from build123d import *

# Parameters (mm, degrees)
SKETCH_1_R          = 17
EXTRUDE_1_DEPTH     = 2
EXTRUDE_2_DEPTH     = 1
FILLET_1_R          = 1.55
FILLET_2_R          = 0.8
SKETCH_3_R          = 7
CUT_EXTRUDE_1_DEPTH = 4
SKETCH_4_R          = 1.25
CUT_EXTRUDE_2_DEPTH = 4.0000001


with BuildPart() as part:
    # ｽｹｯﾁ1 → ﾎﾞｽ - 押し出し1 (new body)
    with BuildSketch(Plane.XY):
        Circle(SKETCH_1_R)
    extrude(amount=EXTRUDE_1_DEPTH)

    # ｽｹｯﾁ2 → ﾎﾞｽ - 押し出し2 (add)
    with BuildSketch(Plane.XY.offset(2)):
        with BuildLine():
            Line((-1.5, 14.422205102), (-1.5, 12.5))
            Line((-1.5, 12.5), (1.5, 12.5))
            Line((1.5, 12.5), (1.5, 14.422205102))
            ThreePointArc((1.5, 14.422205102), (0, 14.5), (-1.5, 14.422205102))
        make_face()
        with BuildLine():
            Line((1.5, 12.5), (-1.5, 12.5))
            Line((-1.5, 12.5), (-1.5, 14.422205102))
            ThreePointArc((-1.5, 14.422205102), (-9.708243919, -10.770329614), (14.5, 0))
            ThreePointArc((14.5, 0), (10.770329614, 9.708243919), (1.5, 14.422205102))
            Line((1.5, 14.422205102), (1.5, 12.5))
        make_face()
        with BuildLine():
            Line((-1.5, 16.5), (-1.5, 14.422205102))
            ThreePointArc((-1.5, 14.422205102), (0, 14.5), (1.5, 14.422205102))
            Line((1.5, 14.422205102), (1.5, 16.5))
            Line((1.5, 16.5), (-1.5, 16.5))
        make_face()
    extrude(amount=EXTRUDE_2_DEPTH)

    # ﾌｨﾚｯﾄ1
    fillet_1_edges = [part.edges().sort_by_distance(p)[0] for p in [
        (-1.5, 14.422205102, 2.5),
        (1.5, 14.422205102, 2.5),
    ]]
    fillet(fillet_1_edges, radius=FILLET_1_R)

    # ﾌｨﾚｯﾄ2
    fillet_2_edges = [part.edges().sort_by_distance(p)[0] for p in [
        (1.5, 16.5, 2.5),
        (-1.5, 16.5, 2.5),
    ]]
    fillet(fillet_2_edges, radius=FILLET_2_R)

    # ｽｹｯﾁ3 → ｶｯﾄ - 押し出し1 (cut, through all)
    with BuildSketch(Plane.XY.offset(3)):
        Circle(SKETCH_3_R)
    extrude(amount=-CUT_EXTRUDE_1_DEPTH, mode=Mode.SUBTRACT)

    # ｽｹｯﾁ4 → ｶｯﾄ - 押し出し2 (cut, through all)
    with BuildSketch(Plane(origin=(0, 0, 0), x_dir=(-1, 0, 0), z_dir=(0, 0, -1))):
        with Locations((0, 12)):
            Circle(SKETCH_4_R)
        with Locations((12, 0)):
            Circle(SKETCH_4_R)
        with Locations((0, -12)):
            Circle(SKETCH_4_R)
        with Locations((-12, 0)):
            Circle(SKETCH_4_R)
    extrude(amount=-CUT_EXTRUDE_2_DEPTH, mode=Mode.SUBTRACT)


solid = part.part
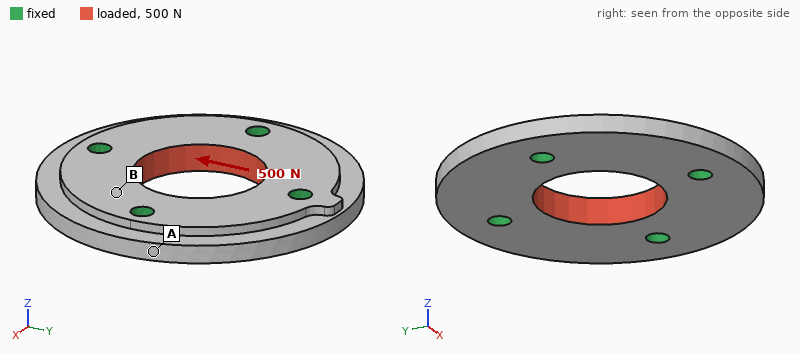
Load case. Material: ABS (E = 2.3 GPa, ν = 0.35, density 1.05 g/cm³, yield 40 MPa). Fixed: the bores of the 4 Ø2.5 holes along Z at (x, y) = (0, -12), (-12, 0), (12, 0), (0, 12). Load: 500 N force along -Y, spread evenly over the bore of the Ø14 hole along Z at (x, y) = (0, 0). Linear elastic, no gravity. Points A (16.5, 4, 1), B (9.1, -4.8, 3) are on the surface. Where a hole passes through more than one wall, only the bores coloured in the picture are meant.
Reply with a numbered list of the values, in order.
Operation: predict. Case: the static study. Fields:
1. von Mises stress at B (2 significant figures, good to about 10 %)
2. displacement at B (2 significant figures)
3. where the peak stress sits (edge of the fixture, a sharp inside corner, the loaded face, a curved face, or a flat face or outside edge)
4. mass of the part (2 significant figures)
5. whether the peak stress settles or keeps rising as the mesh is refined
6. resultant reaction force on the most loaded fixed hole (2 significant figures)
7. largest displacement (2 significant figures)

1. 2.8 MPa
2. 14 µm
3. edge of the fixture
4. 2.1 g
5. keeps rising
6. 130 N
7. 23 µm
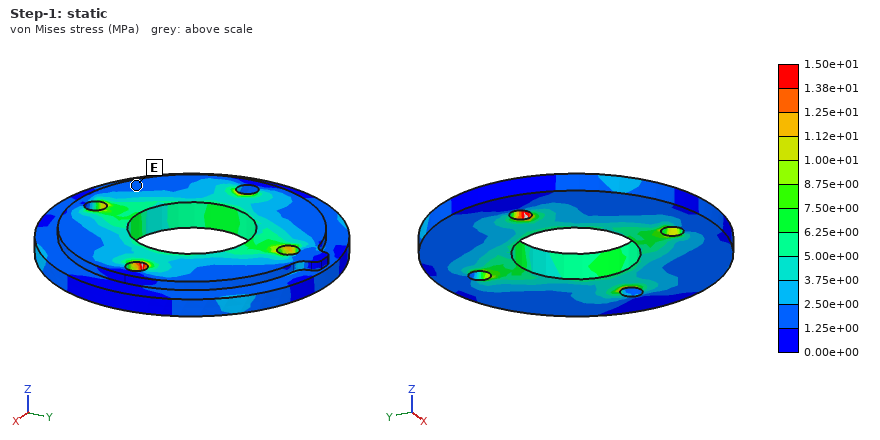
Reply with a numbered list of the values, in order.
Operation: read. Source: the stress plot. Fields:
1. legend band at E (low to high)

1. 1.25e+00 to 2.50e+00 MPa
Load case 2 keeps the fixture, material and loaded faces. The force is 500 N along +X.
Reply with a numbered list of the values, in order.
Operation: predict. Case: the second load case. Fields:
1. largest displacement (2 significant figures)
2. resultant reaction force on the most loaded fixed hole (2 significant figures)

1. 23 µm
2. 130 N
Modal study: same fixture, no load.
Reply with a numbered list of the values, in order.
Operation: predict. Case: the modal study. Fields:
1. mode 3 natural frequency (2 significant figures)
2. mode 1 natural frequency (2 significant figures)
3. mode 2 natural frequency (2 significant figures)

1. 9100 Hz
2. 8700 Hz
3. 9000 Hz
